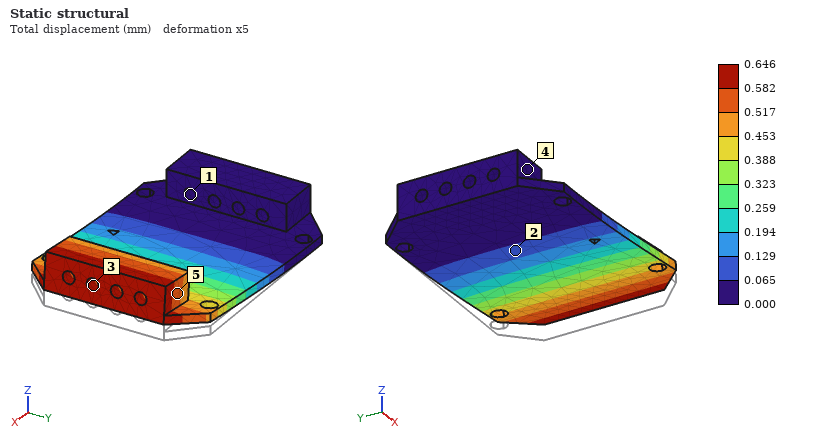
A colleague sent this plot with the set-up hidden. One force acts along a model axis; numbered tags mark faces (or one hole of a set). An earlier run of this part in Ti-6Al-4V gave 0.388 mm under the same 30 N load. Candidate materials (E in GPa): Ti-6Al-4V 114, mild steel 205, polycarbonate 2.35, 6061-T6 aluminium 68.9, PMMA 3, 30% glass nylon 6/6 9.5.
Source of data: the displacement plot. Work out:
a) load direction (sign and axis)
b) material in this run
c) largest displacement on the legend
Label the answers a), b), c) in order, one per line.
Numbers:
a) +Z
b) 6061-T6 aluminium
c) 0.646 mm
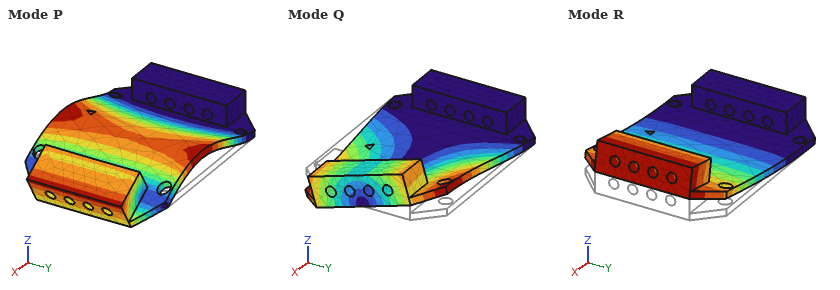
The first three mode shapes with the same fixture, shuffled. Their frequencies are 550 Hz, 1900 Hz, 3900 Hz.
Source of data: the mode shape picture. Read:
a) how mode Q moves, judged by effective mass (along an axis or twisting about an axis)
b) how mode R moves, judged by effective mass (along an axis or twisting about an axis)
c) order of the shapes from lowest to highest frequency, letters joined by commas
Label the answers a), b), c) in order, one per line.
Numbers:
a) twisting about X
b) along Z
c) R, Q, P
